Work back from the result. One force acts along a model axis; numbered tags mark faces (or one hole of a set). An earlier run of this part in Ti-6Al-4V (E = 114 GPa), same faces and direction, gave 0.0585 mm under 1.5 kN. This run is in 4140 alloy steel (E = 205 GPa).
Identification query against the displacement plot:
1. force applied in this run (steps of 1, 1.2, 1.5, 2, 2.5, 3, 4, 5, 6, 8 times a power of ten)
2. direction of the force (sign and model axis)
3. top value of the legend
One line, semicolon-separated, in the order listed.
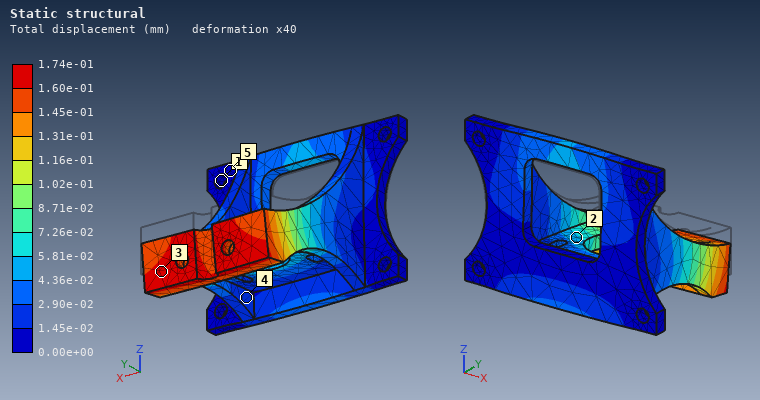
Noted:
8 kN; -Z; 1.74e-01 mm
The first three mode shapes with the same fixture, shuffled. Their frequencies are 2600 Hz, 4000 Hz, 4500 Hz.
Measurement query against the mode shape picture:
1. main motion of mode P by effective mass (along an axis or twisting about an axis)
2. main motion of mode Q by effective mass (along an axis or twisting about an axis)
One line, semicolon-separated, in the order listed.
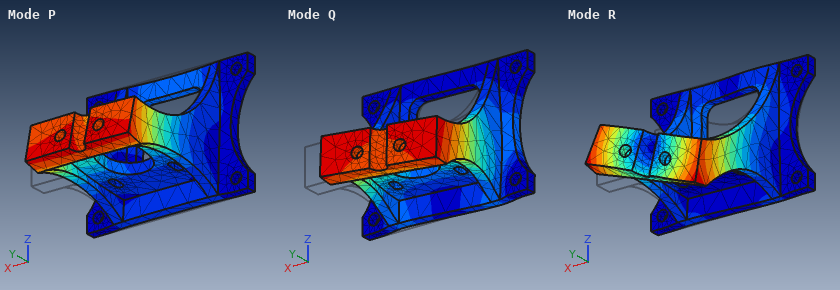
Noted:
along Z; along X
